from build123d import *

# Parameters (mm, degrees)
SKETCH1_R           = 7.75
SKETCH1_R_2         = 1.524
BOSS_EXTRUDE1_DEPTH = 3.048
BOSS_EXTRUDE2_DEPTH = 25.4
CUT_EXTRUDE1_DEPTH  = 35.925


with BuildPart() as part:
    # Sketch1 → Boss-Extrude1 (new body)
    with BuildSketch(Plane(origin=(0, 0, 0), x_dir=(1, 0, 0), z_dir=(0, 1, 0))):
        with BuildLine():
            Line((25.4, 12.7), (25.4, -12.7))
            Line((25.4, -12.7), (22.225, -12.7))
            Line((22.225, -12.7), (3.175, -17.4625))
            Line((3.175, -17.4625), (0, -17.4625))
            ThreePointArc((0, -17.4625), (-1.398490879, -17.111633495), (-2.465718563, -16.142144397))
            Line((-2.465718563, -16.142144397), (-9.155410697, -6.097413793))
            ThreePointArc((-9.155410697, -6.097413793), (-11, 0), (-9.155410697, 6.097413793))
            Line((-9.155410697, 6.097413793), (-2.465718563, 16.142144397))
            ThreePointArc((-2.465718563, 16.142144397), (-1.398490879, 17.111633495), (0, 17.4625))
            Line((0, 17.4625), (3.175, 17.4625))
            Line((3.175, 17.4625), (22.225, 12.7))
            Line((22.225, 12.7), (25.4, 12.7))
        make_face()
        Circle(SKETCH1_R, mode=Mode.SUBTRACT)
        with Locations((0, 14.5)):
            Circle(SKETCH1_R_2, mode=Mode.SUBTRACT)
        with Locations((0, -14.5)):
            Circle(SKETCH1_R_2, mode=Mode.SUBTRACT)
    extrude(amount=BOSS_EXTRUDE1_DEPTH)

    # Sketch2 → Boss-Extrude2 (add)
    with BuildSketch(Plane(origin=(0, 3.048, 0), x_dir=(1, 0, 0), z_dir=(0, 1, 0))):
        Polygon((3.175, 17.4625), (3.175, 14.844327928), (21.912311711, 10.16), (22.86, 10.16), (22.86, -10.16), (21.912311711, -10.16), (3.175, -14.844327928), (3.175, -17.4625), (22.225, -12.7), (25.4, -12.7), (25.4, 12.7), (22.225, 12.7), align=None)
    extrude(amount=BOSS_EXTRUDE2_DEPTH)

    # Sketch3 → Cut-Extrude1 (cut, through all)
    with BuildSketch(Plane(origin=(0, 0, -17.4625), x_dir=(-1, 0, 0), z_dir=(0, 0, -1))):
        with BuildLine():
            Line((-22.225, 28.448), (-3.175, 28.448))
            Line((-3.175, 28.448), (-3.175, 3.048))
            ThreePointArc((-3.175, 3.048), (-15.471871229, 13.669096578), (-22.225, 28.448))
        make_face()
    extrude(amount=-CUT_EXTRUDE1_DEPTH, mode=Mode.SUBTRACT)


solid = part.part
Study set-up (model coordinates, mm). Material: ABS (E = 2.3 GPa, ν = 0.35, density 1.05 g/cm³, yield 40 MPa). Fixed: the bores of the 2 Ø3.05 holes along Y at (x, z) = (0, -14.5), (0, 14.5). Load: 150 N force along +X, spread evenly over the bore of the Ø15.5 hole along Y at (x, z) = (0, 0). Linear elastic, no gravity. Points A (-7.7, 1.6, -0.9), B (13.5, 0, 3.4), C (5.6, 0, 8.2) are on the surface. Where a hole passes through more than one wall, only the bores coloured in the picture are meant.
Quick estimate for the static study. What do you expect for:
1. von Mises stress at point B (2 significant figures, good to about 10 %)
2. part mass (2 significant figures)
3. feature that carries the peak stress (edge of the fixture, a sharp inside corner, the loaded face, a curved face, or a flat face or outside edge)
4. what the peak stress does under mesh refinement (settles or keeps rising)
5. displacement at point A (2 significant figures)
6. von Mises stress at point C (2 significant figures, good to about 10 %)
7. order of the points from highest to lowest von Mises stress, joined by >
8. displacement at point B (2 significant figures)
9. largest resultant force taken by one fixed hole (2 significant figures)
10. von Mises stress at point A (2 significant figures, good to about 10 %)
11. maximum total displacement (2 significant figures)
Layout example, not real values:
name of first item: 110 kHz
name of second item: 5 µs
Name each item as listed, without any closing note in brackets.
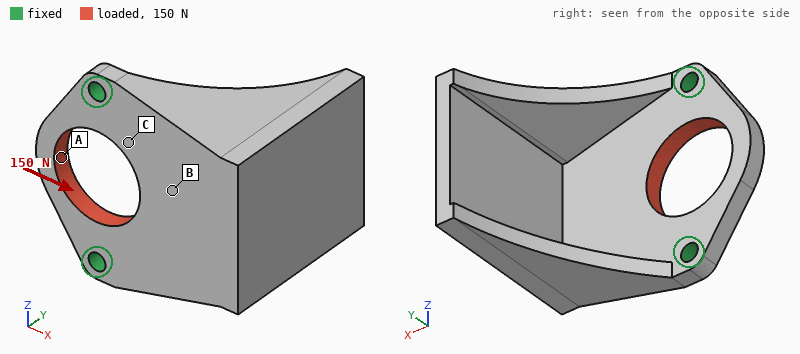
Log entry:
von Mises stress at point B: 0.85 MPa
part mass: 5.3 g
feature that carries the peak stress: edge of the fixture
what the peak stress does under mesh refinement: keeps rising
displacement at point A: 33 µm
von Mises stress at point C: 1.6 MPa
order of the points from highest to lowest von Mises stress, joined by >: A > C > B
displacement at point B: 14 µm
largest resultant force taken by one fixed hole: 75 N
von Mises stress at point A: 2.6 MPa
maximum total displacement: 33 µm
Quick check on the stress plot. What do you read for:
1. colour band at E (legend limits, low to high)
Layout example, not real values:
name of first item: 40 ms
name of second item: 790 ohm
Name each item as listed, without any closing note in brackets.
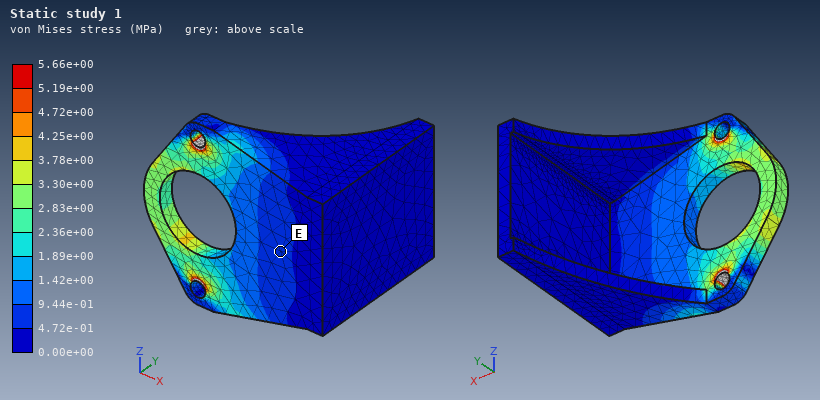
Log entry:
colour band at E: 4.72e-01 to 9.44e-01 MPa
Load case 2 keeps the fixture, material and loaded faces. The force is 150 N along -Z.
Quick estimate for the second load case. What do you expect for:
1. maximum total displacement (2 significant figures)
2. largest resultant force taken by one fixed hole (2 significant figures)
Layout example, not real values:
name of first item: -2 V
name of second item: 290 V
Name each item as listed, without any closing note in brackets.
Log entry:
maximum total displacement: 30 µm
largest resultant force taken by one fixed hole: 75 N
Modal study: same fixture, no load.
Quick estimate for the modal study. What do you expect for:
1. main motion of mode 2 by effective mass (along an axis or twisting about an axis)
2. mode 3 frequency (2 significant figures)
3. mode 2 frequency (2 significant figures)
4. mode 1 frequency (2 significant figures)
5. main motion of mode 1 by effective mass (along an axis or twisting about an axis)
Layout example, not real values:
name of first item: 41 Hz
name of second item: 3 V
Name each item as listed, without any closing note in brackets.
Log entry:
main motion of mode 2 by effective mass: along Z
mode 3 frequency: 3000 Hz
mode 2 frequency: 1100 Hz
mode 1 frequency: 460 Hz
main motion of mode 1 by effective mass: along Y
